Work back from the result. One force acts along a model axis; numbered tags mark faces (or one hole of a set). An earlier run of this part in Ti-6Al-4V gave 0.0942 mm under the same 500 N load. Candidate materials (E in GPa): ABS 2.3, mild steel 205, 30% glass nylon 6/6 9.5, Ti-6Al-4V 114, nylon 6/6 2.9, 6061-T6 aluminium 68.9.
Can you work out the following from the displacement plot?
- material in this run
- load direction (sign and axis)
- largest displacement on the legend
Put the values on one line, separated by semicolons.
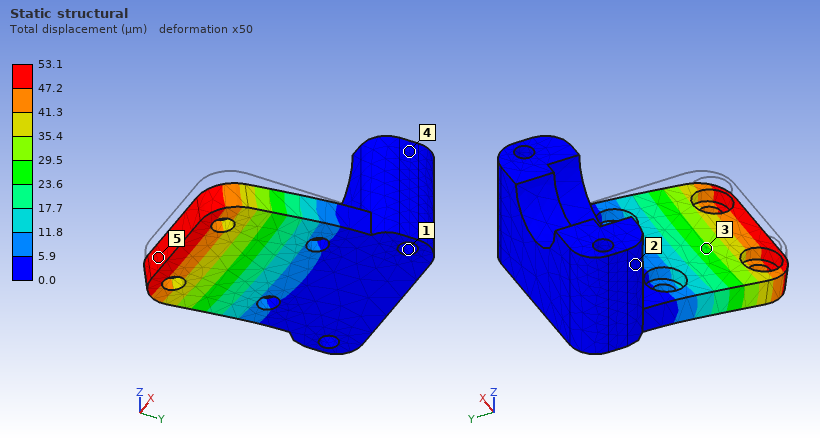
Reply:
mild steel; -Z; 53.1 µm
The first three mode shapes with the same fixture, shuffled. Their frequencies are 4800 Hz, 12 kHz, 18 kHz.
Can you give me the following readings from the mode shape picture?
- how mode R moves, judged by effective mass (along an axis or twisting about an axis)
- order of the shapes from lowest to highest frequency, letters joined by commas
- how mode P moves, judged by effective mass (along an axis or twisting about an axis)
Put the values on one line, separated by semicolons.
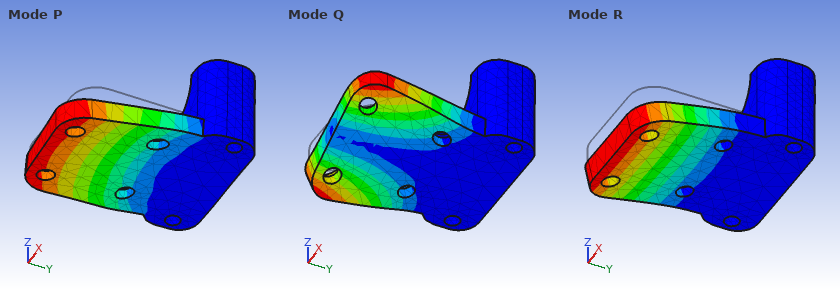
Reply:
along Z; R, Q, P; along X
